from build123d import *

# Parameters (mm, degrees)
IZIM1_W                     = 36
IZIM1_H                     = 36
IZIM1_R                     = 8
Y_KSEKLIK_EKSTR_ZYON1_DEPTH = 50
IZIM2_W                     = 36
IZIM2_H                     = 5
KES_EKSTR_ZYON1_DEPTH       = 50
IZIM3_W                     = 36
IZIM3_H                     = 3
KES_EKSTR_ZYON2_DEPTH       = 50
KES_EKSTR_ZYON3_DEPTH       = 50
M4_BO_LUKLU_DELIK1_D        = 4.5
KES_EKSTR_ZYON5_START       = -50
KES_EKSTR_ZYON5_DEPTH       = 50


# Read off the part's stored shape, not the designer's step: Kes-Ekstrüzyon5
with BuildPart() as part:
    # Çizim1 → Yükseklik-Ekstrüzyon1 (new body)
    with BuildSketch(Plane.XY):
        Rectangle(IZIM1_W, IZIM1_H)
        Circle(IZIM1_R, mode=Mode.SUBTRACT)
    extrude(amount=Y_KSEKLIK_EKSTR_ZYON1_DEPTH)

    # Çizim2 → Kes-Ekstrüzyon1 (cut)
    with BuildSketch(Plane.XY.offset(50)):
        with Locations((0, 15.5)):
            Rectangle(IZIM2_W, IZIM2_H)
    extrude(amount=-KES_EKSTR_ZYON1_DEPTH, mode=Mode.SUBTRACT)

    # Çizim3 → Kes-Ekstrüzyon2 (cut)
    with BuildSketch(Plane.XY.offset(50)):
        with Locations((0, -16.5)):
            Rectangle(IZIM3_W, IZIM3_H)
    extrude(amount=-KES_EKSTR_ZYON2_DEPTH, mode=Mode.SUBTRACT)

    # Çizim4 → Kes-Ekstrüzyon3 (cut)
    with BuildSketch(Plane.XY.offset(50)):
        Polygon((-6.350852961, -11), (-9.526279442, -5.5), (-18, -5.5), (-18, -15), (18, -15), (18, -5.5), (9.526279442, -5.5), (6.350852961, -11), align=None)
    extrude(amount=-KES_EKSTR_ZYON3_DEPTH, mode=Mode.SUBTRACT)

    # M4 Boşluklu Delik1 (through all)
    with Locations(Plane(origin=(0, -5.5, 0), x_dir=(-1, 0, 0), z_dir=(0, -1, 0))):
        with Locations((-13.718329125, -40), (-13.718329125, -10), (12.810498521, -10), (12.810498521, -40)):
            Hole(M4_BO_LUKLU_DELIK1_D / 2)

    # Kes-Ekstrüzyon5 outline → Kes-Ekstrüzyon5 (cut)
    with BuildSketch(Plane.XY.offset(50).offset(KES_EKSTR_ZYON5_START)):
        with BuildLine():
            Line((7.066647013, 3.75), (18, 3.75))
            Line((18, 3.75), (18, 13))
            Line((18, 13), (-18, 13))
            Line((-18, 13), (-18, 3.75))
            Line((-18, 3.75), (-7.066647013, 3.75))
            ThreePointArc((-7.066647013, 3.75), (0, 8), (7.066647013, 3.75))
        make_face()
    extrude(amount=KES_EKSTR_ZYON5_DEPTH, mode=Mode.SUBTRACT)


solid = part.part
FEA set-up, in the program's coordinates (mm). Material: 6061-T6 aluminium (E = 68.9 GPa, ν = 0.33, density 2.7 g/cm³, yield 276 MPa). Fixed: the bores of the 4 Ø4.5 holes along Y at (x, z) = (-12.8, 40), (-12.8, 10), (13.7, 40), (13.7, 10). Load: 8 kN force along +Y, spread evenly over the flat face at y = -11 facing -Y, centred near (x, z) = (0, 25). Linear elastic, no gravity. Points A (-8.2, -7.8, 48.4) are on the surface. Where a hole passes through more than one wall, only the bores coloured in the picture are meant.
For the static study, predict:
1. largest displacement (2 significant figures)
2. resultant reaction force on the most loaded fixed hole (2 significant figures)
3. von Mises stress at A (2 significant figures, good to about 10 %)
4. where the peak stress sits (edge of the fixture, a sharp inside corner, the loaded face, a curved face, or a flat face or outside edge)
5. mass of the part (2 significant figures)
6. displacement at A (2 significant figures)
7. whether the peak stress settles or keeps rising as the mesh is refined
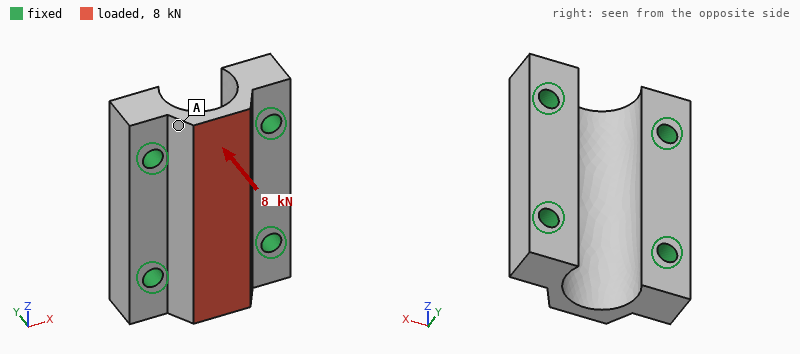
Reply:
16 µm
2.7 kN
8.7 MPa
edge of the fixture
34 g
5.0 µm
keeps rising
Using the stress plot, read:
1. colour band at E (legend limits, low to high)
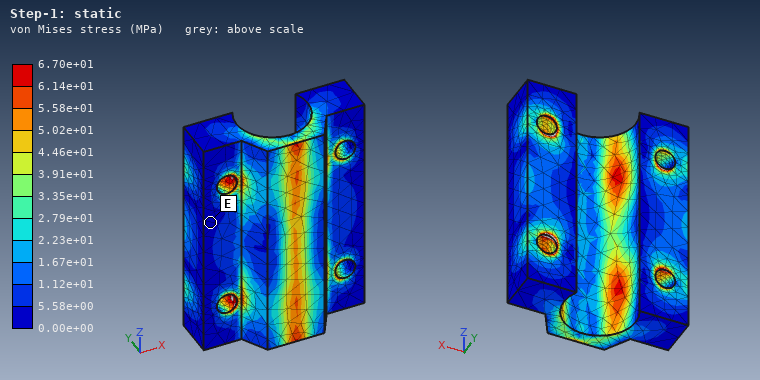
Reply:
0.00e+00 to 5.58e+00 MPa
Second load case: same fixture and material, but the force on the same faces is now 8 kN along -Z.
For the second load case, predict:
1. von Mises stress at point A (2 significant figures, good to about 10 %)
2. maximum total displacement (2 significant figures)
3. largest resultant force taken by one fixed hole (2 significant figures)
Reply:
27 MPa
27 µm
2.4 kN
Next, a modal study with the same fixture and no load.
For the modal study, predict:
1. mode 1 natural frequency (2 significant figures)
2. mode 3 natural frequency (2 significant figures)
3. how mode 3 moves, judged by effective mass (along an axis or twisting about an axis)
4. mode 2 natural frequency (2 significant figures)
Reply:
35 kHz
38 kHz
along Z
36 kHz
